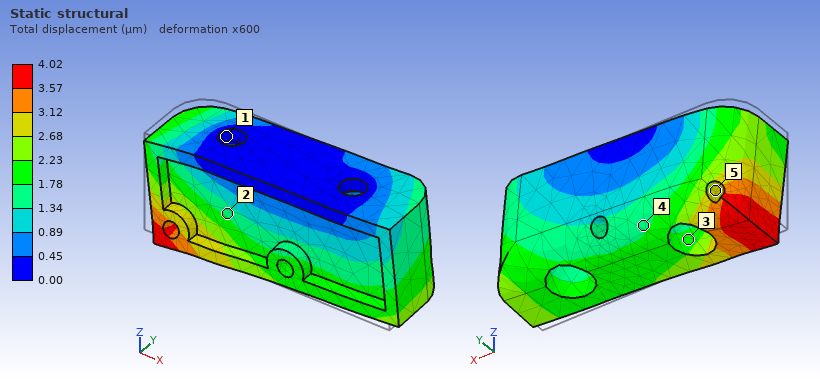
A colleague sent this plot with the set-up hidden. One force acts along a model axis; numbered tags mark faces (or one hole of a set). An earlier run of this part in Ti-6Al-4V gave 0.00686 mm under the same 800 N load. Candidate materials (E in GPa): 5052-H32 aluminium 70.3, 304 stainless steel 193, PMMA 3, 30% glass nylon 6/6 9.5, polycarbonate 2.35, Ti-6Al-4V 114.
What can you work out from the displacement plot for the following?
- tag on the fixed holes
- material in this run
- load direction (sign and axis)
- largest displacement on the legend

1
304 stainless steel
+X
4.02 µm
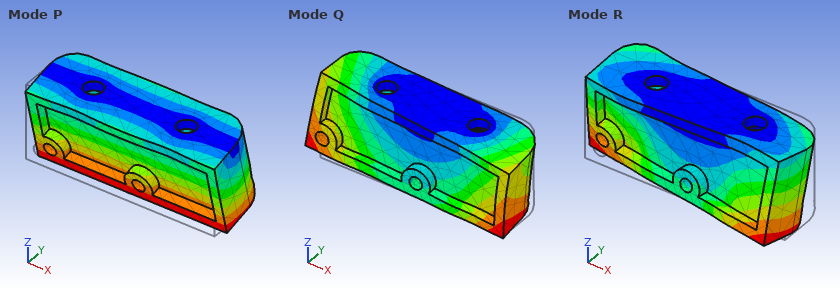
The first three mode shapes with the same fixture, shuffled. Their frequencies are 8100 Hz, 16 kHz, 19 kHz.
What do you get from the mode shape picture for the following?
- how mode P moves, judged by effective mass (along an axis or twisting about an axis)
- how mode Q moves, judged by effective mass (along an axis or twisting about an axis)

along Y
along X
